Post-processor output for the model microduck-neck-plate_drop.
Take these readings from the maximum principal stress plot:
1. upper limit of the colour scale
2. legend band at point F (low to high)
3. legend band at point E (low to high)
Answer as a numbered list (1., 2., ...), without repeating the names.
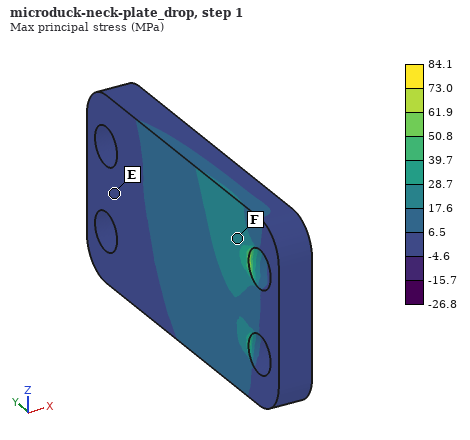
1. 84.1 MPa
2. 17.6 to 28.7 MPa
3. -4.6 to 6.5 MPa
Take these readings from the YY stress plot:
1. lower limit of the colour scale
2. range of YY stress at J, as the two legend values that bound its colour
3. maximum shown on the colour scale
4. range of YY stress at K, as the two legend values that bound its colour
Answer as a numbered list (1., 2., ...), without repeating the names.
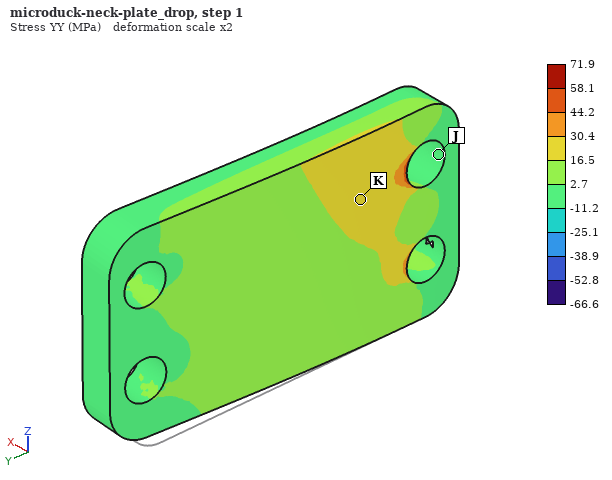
1. -66.6 MPa
2. -11.2 to 2.7 MPa
3. 71.9 MPa
4. 16.5 to 30.4 MPa
